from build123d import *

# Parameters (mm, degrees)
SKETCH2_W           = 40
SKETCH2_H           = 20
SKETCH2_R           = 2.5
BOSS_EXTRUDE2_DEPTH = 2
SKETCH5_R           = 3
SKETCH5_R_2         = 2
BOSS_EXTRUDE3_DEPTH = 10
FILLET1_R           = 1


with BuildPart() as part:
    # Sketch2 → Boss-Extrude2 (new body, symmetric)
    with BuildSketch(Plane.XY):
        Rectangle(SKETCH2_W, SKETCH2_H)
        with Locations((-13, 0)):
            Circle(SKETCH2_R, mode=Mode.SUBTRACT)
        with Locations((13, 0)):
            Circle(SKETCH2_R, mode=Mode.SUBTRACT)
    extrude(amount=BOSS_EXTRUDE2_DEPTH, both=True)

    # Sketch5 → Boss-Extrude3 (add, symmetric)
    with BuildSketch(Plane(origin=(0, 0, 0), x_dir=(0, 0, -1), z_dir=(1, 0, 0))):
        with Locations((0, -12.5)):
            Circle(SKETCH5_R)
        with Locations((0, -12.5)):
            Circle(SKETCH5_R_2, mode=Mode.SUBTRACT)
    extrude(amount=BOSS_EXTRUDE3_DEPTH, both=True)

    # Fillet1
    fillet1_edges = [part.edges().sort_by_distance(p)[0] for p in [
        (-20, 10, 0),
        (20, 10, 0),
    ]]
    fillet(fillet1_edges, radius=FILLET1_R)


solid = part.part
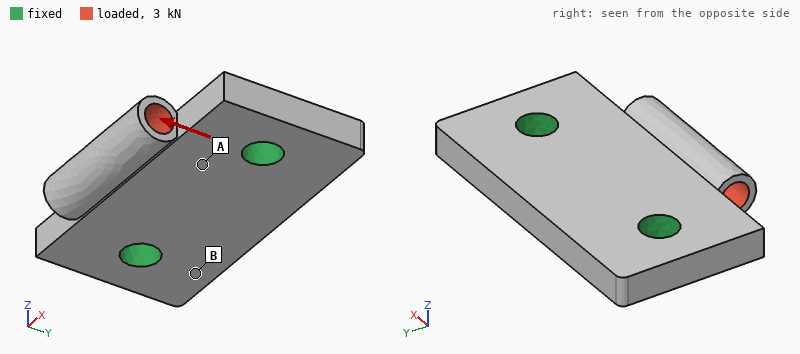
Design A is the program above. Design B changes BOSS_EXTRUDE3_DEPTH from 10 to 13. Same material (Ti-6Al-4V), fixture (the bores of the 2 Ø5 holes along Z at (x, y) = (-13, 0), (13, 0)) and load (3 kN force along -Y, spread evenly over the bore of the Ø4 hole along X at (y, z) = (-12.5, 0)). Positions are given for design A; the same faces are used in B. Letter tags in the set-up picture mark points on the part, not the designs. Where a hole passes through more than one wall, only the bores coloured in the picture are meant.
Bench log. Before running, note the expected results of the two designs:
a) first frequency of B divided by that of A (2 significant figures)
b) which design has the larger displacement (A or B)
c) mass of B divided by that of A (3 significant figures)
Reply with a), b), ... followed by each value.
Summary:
a) 0.98
b) A
c) 1.03
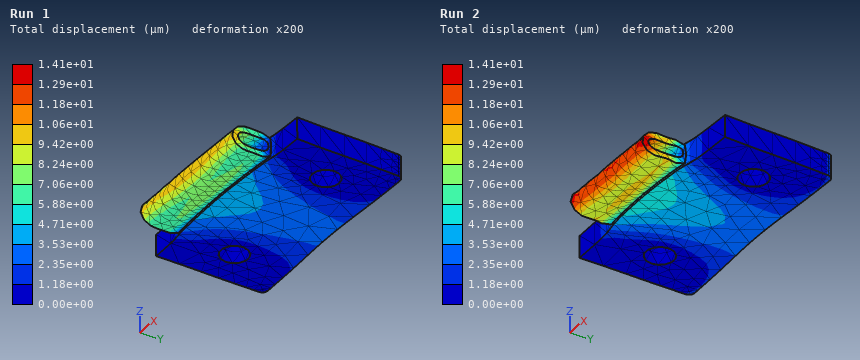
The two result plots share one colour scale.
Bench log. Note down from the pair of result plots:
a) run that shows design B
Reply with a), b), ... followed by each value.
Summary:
a) Run 1
